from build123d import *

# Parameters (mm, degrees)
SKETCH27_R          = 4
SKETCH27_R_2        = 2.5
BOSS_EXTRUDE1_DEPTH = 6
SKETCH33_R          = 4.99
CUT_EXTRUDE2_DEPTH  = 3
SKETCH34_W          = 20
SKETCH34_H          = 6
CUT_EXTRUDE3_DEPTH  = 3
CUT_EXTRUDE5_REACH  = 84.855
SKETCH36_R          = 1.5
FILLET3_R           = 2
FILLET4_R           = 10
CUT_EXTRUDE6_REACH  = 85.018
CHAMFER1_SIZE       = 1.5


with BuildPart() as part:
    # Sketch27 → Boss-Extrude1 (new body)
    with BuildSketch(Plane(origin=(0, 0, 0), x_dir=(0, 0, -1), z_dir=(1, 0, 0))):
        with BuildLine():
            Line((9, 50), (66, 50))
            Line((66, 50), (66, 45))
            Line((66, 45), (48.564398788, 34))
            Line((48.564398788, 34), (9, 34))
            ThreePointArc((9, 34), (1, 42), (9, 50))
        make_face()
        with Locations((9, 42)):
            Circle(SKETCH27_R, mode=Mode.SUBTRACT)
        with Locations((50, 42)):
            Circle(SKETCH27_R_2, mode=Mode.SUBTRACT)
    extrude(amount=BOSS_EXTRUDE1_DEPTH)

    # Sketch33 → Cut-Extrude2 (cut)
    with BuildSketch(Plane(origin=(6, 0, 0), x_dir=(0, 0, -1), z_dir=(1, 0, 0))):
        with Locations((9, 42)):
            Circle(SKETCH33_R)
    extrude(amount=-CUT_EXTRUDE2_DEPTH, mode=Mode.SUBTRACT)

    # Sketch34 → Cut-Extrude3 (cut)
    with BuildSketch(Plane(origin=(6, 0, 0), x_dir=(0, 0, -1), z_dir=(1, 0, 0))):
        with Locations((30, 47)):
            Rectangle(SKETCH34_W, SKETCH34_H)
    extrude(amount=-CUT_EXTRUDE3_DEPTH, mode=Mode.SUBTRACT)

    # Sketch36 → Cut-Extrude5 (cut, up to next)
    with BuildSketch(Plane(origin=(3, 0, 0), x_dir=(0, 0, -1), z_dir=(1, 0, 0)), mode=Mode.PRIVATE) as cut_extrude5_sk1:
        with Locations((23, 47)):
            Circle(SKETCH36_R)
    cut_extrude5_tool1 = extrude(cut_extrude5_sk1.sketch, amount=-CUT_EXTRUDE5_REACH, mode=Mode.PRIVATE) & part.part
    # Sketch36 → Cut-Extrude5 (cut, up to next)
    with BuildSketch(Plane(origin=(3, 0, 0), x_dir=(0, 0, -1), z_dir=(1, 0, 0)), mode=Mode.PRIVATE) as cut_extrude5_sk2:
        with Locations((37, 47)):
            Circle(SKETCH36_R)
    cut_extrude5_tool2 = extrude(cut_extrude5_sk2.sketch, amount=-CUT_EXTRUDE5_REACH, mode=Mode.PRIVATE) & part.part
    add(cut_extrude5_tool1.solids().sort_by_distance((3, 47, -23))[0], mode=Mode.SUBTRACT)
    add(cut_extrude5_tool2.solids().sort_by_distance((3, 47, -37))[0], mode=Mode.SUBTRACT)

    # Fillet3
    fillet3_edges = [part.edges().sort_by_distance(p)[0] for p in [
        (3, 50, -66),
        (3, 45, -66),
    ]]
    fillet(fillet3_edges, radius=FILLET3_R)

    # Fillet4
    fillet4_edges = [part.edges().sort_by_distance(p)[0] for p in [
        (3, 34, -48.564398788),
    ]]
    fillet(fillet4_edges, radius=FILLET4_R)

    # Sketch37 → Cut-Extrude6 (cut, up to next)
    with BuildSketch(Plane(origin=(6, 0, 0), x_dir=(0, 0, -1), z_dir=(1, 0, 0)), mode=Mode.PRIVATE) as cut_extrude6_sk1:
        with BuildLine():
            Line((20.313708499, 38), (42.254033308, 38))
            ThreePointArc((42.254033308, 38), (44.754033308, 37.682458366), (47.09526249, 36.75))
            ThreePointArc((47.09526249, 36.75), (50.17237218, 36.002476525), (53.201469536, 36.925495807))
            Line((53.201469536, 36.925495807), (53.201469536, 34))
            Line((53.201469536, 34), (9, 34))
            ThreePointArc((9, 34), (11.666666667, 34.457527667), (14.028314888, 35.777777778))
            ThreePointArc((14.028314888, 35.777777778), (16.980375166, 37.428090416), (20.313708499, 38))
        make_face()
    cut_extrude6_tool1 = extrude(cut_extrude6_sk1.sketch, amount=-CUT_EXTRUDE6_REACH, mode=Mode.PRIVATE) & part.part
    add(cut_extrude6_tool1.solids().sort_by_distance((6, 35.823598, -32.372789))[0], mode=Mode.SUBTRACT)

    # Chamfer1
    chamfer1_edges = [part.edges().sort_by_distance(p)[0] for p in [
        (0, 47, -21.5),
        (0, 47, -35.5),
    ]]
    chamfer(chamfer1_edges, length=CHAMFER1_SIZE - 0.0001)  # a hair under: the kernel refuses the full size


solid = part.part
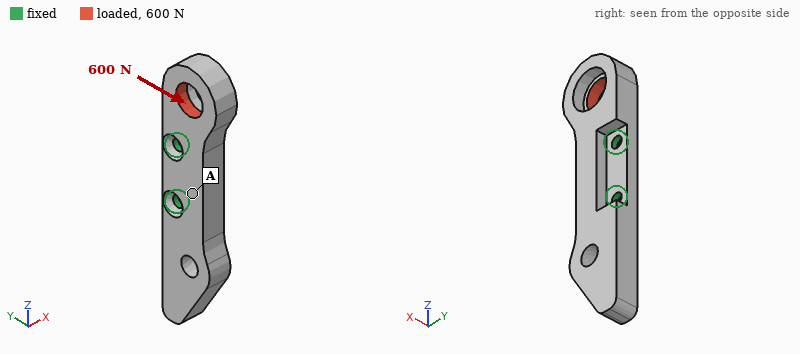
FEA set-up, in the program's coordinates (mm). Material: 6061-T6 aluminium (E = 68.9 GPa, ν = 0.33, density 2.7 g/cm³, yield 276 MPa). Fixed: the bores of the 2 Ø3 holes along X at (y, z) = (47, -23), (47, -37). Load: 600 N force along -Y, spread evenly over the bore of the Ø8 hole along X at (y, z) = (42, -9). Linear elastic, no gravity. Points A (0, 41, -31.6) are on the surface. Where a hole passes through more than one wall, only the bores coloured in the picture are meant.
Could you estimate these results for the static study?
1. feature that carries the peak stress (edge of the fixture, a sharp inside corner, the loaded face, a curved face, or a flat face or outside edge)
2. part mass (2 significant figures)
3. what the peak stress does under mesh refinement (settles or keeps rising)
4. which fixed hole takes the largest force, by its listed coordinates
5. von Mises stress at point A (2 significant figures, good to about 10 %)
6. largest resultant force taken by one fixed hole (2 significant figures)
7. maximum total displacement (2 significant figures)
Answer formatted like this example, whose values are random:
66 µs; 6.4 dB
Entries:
edge of the fixture; 10 g; keeps rising; (47, -23); 25 MPa; 1.1 kN; 72 µm
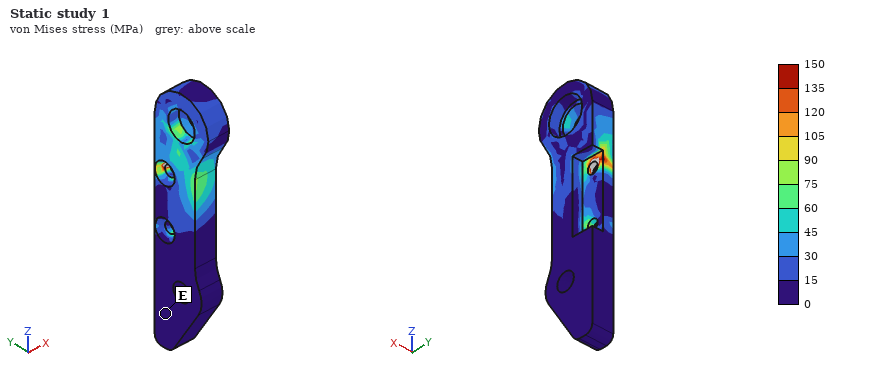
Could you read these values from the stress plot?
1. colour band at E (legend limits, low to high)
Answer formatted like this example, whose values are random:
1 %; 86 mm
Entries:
0 to 15 MPa
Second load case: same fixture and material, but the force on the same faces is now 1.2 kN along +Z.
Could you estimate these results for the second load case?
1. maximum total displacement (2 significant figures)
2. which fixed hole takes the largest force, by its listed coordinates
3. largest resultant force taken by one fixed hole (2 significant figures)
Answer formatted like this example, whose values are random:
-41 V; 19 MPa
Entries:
61 µm; (47, -23); 830 N
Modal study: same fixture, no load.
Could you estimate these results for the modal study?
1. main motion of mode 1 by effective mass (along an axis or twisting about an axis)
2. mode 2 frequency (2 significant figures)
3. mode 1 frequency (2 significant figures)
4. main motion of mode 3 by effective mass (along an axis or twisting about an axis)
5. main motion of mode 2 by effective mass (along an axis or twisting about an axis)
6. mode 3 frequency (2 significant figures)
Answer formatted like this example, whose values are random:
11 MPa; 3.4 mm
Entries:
along X; 5600 Hz; 3900 Hz; along Y; along X; 8000 Hz
